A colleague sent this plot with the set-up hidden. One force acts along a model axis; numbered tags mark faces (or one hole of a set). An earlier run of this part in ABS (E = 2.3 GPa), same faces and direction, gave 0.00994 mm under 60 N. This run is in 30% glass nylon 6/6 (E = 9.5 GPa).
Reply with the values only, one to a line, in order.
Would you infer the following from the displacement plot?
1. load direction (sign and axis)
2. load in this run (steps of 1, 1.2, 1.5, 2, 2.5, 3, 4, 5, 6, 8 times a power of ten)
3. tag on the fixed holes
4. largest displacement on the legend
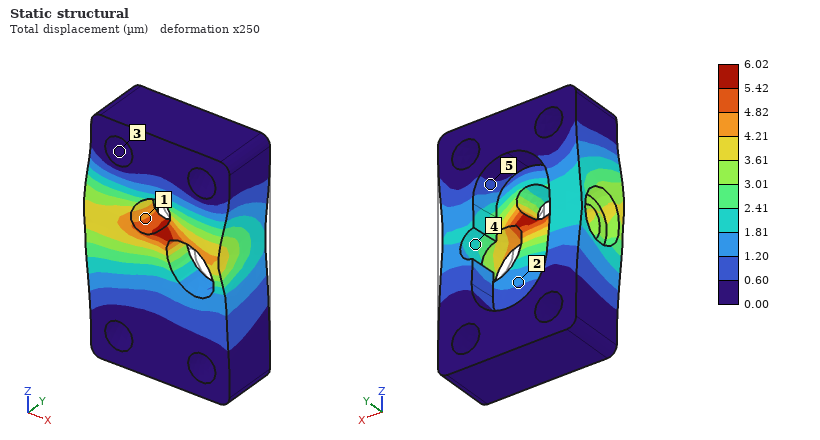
-X
150 N
3
6.02 µm
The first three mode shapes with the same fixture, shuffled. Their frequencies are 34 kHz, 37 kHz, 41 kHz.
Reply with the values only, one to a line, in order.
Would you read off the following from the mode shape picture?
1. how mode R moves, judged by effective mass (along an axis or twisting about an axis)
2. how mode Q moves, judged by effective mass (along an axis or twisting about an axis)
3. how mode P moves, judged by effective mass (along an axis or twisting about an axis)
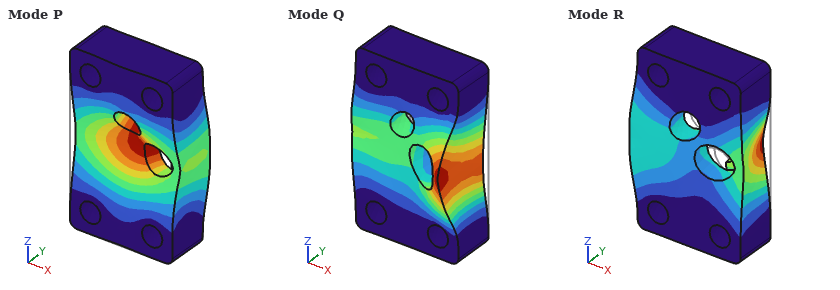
along X
along X
along Y
